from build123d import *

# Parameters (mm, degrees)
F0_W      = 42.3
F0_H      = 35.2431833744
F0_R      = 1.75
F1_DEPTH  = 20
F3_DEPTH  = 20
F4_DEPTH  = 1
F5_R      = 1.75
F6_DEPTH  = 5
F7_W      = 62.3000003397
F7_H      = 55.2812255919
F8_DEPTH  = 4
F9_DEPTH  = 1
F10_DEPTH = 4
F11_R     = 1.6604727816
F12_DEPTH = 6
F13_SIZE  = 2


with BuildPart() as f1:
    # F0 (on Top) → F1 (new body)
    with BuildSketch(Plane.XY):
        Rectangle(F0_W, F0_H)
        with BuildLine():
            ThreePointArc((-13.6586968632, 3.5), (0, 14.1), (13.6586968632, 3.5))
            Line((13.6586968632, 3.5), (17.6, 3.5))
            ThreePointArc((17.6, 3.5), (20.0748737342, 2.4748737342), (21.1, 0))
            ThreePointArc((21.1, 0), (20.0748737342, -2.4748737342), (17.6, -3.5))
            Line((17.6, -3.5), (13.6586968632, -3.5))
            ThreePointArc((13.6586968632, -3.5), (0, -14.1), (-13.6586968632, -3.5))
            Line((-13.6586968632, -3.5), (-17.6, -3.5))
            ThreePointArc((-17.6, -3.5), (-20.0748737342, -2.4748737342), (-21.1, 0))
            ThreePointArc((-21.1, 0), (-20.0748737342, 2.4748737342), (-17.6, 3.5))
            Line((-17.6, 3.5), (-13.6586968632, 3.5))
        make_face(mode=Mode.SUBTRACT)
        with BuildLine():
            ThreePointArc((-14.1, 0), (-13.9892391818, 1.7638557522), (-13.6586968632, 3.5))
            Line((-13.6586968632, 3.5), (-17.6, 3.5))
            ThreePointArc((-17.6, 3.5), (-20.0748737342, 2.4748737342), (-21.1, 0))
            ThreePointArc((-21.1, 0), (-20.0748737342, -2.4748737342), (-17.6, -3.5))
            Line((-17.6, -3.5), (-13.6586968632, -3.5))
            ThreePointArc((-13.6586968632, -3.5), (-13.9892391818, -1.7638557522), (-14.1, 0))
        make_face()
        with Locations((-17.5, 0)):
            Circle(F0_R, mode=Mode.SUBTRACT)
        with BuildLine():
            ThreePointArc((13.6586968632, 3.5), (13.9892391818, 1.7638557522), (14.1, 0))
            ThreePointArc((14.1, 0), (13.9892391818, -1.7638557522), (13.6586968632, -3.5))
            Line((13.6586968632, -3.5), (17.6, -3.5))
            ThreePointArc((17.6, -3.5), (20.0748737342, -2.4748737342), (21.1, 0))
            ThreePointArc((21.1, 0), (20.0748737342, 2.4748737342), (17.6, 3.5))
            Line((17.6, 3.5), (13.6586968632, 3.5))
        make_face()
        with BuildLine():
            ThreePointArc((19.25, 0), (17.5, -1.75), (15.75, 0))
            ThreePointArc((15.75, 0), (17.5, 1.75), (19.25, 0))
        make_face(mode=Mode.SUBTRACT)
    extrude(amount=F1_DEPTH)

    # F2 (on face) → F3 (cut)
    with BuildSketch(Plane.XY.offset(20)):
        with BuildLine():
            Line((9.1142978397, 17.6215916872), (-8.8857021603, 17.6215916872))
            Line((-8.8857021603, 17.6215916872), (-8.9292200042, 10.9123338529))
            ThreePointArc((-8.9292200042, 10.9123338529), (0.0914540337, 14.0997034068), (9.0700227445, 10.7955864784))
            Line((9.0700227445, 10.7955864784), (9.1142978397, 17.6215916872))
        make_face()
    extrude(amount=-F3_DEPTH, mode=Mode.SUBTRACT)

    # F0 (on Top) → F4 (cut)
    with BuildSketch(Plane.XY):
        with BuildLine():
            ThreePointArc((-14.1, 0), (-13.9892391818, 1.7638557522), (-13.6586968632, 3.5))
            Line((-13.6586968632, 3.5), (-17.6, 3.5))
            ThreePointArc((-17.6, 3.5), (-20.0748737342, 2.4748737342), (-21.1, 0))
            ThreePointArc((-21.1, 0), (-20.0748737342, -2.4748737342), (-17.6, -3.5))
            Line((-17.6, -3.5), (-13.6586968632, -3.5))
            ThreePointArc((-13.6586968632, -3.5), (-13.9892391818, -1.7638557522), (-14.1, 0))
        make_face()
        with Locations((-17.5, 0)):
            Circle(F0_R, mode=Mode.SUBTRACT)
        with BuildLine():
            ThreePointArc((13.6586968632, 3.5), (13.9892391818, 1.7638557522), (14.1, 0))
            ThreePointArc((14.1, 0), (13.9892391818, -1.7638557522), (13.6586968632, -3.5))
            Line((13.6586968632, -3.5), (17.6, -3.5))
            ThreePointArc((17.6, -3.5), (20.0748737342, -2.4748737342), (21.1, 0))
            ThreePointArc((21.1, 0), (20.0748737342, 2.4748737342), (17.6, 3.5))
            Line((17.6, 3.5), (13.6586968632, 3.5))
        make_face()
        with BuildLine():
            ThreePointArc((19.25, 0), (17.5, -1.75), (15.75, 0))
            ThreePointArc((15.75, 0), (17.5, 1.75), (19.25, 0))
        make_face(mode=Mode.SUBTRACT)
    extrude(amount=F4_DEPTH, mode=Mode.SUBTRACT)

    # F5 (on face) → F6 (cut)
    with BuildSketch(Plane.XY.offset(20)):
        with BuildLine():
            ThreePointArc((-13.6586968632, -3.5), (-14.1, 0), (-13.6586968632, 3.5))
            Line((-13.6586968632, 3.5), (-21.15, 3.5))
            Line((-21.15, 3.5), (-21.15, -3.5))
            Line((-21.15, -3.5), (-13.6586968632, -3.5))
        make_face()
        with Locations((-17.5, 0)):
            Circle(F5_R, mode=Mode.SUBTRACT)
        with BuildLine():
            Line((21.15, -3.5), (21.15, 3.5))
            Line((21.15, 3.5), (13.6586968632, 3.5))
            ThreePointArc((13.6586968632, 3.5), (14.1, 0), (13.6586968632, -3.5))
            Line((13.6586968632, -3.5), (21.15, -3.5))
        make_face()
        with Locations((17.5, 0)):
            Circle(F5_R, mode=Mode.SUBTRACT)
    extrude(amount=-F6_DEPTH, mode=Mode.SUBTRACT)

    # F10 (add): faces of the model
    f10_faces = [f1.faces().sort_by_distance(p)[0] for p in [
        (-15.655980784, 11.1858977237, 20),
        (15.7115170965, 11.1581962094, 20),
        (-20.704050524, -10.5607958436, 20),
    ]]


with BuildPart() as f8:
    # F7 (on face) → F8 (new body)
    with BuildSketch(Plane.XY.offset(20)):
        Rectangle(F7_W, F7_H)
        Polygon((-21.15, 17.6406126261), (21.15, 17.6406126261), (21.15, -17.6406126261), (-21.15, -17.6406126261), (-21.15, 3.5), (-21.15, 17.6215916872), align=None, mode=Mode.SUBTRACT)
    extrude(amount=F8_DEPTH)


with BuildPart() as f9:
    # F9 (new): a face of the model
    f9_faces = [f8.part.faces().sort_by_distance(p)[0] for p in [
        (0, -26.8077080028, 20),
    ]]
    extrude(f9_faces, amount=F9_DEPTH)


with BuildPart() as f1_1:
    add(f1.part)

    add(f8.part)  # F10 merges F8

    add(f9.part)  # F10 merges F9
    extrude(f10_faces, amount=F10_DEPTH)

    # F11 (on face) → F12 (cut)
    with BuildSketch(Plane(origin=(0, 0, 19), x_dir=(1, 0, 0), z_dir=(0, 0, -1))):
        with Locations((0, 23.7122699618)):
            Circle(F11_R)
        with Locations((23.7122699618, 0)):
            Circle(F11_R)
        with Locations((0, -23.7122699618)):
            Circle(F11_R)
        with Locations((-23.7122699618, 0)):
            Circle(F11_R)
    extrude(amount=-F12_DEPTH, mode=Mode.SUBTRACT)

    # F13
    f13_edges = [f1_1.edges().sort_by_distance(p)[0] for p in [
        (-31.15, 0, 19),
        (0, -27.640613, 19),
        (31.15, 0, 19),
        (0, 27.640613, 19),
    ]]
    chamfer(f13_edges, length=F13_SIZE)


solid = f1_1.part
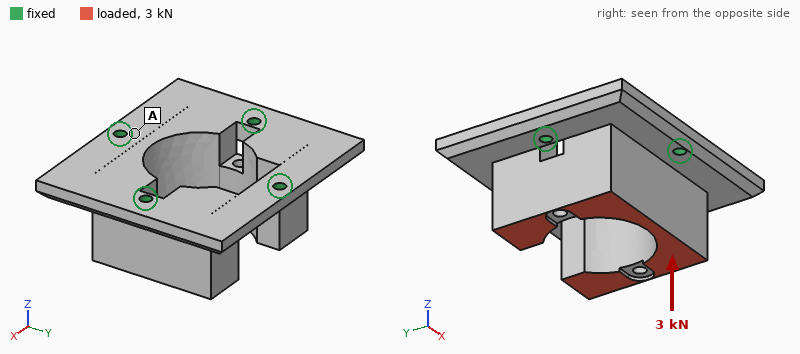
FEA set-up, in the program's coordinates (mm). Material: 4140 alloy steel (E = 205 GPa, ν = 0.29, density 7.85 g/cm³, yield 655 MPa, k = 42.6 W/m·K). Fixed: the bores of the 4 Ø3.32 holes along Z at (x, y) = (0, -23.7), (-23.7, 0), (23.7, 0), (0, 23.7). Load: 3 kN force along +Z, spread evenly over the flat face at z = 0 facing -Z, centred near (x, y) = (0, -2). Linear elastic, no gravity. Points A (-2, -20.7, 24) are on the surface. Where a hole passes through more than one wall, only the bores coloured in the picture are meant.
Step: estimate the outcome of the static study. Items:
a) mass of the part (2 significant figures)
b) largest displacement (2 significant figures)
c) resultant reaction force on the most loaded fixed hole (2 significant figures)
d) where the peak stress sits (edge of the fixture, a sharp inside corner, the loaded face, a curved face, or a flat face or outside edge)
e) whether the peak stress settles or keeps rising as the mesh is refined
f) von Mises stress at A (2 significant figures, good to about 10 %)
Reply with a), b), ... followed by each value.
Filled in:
a) 210 g
b) 13 µm
c) 1.4 kN
d) a sharp inside corner
e) keeps rising
f) 20 MPa
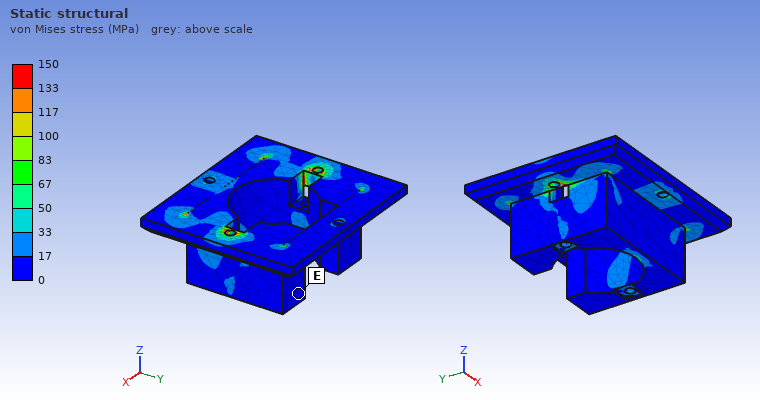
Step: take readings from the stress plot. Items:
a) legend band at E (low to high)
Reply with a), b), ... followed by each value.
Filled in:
a) 0 to 17 MPa
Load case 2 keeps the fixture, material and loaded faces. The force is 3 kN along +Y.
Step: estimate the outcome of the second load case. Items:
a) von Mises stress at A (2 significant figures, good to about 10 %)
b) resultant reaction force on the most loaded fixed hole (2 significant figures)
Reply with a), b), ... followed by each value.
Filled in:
a) 75 MPa
b) 1.4 kN
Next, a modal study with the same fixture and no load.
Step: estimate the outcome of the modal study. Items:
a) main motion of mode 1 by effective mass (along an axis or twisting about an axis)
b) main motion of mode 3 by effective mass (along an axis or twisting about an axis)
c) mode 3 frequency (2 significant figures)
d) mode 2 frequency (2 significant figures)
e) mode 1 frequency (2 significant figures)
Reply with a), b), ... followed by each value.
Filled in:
a) along Y
b) along Z
c) 6800 Hz
d) 5100 Hz
e) 4600 Hz
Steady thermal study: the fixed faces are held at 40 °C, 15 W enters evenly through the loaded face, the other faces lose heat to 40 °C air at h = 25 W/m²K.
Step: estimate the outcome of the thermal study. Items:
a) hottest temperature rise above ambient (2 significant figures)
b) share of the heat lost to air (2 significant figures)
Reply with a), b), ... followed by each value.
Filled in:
a) 23 K
b) 21 %
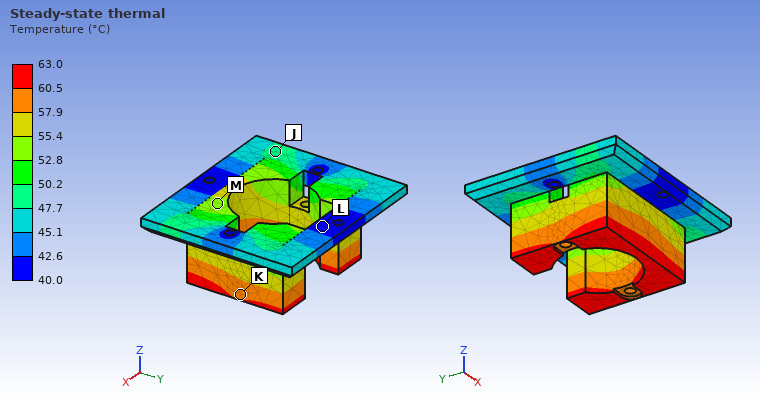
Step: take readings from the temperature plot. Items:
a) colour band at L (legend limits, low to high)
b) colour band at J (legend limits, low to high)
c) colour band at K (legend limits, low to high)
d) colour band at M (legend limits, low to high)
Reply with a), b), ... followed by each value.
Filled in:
a) 40.0 to 42.6 °C
b) 47.7 to 50.2 °C
c) 57.9 to 60.5 °C
d) 52.8 to 55.4 °C
